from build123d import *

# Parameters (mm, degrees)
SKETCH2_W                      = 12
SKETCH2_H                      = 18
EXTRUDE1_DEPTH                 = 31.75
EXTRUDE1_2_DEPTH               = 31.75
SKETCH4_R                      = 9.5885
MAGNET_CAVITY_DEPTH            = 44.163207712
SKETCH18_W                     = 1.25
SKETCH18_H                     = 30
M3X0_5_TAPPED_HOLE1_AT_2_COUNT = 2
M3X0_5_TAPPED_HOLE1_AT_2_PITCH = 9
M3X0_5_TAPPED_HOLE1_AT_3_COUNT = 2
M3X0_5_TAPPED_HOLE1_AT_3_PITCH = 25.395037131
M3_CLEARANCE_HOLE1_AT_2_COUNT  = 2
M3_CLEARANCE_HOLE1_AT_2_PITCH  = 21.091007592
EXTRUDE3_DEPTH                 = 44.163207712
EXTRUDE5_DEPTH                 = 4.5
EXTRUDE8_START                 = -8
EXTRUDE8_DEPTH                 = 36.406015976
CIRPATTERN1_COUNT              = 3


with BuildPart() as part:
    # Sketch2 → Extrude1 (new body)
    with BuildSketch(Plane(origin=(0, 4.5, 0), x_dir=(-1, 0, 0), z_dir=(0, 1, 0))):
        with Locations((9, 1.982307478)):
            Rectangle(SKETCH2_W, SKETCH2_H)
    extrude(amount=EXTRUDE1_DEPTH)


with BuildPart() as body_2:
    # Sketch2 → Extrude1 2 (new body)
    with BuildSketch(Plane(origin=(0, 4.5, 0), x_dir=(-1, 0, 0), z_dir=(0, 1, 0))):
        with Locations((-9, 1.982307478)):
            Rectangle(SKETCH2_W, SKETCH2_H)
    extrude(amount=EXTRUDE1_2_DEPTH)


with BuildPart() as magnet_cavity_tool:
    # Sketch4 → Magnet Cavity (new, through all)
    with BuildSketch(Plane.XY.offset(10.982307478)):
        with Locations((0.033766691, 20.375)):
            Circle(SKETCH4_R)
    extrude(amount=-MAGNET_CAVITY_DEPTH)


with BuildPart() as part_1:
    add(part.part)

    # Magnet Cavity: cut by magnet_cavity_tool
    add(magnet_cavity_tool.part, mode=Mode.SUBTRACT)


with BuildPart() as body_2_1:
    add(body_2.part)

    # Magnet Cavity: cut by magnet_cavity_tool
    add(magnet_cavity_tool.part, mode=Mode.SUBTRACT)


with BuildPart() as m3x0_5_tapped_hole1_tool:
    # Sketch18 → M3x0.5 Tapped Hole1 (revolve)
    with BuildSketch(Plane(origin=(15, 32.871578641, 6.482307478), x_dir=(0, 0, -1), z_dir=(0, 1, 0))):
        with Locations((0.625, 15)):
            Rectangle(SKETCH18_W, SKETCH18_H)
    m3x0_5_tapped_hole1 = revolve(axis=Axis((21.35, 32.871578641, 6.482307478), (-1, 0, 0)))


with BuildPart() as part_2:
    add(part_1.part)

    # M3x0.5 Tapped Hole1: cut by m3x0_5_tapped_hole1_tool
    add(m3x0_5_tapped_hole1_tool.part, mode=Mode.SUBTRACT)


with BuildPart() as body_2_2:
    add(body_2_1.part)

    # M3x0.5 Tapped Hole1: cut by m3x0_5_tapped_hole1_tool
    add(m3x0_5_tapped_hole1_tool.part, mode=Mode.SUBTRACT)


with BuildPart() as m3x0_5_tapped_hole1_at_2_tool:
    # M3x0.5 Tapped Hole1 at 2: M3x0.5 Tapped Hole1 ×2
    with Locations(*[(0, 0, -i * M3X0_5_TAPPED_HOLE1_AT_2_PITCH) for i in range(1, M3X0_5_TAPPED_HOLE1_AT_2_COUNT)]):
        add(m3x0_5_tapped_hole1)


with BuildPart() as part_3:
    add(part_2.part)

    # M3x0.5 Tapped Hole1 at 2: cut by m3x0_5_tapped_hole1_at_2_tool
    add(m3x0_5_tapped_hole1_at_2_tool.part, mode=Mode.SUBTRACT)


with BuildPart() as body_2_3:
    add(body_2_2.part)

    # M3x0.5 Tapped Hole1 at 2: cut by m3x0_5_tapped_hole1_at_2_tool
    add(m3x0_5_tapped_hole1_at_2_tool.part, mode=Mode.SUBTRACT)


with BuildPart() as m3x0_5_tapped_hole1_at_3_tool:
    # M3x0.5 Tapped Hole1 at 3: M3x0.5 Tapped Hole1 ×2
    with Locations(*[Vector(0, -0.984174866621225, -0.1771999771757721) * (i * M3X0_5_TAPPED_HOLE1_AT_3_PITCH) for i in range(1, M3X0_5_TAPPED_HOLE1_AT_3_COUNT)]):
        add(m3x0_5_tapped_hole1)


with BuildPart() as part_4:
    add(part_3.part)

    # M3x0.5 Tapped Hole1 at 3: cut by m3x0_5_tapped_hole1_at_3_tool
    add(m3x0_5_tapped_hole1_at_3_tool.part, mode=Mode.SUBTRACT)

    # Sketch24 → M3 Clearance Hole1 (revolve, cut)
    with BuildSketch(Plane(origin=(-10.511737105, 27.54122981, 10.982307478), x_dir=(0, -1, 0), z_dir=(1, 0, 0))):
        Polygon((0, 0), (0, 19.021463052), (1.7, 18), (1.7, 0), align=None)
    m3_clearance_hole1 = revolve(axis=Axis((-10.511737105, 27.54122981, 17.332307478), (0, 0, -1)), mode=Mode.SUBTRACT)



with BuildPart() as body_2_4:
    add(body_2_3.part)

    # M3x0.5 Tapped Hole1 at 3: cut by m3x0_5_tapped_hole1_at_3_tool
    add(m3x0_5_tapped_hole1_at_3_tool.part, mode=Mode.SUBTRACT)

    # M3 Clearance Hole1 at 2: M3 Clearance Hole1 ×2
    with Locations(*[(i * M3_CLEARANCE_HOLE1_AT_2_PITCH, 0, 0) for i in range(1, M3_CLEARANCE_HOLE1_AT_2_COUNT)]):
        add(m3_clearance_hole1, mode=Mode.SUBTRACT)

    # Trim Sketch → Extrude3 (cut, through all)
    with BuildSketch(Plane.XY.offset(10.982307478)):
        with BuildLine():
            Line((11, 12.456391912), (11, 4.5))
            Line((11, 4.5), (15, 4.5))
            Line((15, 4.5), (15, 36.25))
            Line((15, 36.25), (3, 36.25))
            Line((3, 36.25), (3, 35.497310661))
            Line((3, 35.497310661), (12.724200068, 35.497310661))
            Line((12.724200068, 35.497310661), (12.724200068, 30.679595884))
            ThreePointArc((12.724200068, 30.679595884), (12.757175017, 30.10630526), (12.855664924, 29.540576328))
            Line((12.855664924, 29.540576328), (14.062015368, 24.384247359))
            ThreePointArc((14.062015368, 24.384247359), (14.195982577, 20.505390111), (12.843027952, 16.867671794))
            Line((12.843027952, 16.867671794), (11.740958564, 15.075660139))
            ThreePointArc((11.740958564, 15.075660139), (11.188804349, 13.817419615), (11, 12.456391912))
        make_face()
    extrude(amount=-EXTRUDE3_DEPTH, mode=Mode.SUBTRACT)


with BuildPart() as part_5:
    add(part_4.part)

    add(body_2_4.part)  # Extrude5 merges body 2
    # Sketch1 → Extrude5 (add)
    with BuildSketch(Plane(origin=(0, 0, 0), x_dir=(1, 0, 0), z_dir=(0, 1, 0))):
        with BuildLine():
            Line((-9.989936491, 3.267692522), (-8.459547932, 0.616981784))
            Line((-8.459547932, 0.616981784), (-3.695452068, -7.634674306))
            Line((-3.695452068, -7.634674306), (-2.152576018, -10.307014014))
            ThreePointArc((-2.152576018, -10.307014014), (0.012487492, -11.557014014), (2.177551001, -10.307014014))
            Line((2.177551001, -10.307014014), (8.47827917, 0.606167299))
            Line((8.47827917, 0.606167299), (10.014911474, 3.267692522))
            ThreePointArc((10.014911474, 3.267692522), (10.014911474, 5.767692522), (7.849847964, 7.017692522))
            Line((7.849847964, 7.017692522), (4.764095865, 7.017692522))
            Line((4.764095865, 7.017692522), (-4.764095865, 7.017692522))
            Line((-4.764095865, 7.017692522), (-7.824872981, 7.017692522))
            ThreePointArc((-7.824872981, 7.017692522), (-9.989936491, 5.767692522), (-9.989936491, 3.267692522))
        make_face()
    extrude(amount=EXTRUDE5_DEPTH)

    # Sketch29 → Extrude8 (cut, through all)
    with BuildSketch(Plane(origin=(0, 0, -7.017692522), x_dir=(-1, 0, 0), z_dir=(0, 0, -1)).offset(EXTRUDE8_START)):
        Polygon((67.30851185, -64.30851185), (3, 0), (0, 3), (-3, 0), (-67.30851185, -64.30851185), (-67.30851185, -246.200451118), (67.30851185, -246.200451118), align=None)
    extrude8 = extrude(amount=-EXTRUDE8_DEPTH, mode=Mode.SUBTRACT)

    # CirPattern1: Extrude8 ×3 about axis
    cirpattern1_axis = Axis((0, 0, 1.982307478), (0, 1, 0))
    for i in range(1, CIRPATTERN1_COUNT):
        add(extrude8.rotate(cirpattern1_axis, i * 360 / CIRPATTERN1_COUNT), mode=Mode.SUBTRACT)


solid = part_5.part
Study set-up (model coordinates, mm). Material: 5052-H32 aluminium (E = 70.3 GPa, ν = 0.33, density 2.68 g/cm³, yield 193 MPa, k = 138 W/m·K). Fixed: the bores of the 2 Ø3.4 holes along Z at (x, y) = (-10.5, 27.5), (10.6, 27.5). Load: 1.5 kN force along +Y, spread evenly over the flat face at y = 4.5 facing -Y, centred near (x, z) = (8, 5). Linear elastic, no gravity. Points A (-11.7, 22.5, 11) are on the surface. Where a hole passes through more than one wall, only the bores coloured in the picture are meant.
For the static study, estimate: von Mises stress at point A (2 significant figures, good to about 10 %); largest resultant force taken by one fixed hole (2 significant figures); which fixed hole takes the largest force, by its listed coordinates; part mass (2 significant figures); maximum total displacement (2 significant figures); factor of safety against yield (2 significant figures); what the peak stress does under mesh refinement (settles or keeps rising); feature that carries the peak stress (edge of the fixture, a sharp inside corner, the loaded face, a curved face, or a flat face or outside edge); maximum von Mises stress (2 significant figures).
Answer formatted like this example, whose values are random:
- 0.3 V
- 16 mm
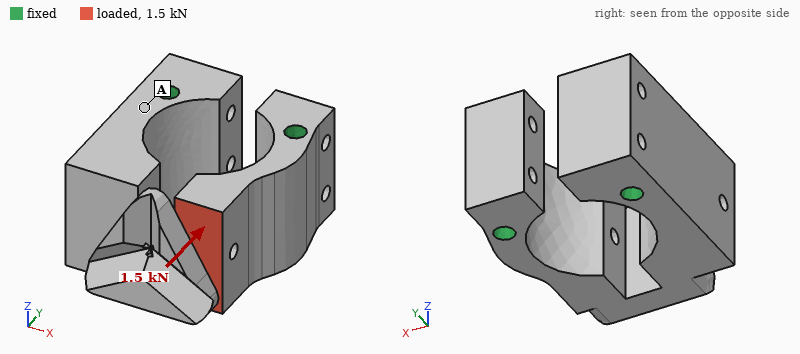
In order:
- 12 MPa
- 1.3 kN
- (10.6, 27.5)
- 25 g
- 23 µm
- 2.3
- settles
- a curved face
- 82 MPa
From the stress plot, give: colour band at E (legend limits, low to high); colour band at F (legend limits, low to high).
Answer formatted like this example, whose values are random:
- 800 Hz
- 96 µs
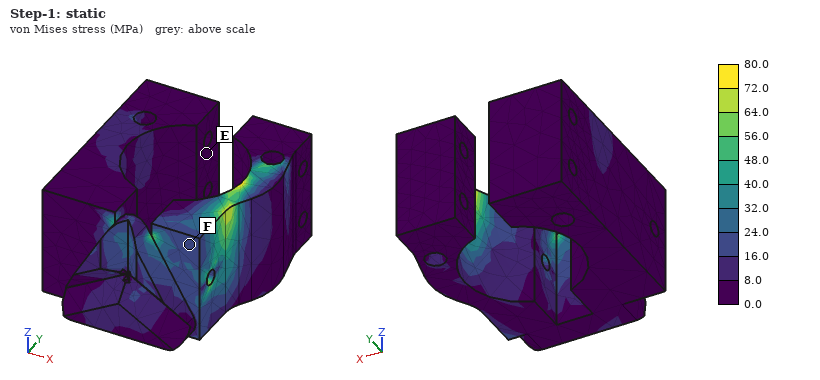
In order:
- 0.0 to 8.0 MPa
- 16.0 to 24.0 MPa
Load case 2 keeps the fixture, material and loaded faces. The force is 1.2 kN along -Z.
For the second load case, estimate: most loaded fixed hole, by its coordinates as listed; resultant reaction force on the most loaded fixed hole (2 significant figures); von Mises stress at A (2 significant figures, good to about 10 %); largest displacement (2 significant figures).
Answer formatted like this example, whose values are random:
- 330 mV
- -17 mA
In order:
- (10.6, 27.5)
- 930 N
- 39 MPa
- 48 µm
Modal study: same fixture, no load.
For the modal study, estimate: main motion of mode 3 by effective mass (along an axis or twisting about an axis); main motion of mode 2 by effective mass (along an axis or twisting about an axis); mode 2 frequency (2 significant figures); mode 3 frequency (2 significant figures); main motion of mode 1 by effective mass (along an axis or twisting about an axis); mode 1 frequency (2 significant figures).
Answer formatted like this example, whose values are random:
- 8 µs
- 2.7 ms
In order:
- twisting about Y
- along Z
- 13 kHz
- 19 kHz
- along X
- 10 kHz
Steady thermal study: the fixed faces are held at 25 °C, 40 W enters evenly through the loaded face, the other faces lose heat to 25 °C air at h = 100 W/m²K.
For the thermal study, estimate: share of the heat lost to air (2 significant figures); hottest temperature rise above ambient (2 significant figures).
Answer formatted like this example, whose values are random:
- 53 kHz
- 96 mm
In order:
- 15 %
- 58 K
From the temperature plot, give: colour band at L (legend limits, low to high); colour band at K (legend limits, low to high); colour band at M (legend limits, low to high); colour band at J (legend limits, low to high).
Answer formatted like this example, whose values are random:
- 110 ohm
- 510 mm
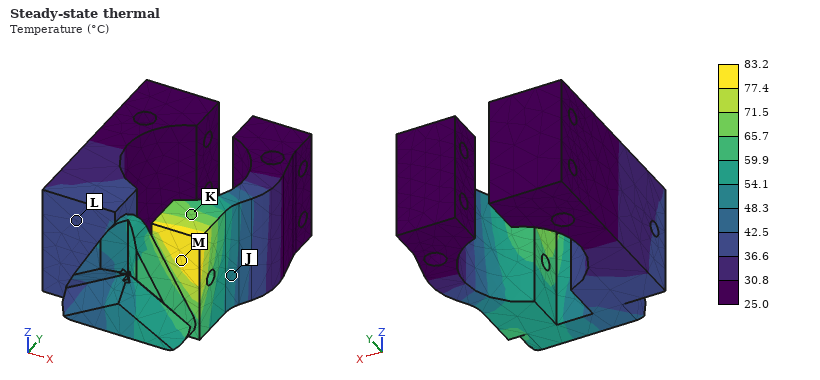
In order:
- 36.6 to 42.5 °C
- 65.7 to 71.5 °C
- 77.4 to 83.2 °C
- 48.3 to 54.1 °C
